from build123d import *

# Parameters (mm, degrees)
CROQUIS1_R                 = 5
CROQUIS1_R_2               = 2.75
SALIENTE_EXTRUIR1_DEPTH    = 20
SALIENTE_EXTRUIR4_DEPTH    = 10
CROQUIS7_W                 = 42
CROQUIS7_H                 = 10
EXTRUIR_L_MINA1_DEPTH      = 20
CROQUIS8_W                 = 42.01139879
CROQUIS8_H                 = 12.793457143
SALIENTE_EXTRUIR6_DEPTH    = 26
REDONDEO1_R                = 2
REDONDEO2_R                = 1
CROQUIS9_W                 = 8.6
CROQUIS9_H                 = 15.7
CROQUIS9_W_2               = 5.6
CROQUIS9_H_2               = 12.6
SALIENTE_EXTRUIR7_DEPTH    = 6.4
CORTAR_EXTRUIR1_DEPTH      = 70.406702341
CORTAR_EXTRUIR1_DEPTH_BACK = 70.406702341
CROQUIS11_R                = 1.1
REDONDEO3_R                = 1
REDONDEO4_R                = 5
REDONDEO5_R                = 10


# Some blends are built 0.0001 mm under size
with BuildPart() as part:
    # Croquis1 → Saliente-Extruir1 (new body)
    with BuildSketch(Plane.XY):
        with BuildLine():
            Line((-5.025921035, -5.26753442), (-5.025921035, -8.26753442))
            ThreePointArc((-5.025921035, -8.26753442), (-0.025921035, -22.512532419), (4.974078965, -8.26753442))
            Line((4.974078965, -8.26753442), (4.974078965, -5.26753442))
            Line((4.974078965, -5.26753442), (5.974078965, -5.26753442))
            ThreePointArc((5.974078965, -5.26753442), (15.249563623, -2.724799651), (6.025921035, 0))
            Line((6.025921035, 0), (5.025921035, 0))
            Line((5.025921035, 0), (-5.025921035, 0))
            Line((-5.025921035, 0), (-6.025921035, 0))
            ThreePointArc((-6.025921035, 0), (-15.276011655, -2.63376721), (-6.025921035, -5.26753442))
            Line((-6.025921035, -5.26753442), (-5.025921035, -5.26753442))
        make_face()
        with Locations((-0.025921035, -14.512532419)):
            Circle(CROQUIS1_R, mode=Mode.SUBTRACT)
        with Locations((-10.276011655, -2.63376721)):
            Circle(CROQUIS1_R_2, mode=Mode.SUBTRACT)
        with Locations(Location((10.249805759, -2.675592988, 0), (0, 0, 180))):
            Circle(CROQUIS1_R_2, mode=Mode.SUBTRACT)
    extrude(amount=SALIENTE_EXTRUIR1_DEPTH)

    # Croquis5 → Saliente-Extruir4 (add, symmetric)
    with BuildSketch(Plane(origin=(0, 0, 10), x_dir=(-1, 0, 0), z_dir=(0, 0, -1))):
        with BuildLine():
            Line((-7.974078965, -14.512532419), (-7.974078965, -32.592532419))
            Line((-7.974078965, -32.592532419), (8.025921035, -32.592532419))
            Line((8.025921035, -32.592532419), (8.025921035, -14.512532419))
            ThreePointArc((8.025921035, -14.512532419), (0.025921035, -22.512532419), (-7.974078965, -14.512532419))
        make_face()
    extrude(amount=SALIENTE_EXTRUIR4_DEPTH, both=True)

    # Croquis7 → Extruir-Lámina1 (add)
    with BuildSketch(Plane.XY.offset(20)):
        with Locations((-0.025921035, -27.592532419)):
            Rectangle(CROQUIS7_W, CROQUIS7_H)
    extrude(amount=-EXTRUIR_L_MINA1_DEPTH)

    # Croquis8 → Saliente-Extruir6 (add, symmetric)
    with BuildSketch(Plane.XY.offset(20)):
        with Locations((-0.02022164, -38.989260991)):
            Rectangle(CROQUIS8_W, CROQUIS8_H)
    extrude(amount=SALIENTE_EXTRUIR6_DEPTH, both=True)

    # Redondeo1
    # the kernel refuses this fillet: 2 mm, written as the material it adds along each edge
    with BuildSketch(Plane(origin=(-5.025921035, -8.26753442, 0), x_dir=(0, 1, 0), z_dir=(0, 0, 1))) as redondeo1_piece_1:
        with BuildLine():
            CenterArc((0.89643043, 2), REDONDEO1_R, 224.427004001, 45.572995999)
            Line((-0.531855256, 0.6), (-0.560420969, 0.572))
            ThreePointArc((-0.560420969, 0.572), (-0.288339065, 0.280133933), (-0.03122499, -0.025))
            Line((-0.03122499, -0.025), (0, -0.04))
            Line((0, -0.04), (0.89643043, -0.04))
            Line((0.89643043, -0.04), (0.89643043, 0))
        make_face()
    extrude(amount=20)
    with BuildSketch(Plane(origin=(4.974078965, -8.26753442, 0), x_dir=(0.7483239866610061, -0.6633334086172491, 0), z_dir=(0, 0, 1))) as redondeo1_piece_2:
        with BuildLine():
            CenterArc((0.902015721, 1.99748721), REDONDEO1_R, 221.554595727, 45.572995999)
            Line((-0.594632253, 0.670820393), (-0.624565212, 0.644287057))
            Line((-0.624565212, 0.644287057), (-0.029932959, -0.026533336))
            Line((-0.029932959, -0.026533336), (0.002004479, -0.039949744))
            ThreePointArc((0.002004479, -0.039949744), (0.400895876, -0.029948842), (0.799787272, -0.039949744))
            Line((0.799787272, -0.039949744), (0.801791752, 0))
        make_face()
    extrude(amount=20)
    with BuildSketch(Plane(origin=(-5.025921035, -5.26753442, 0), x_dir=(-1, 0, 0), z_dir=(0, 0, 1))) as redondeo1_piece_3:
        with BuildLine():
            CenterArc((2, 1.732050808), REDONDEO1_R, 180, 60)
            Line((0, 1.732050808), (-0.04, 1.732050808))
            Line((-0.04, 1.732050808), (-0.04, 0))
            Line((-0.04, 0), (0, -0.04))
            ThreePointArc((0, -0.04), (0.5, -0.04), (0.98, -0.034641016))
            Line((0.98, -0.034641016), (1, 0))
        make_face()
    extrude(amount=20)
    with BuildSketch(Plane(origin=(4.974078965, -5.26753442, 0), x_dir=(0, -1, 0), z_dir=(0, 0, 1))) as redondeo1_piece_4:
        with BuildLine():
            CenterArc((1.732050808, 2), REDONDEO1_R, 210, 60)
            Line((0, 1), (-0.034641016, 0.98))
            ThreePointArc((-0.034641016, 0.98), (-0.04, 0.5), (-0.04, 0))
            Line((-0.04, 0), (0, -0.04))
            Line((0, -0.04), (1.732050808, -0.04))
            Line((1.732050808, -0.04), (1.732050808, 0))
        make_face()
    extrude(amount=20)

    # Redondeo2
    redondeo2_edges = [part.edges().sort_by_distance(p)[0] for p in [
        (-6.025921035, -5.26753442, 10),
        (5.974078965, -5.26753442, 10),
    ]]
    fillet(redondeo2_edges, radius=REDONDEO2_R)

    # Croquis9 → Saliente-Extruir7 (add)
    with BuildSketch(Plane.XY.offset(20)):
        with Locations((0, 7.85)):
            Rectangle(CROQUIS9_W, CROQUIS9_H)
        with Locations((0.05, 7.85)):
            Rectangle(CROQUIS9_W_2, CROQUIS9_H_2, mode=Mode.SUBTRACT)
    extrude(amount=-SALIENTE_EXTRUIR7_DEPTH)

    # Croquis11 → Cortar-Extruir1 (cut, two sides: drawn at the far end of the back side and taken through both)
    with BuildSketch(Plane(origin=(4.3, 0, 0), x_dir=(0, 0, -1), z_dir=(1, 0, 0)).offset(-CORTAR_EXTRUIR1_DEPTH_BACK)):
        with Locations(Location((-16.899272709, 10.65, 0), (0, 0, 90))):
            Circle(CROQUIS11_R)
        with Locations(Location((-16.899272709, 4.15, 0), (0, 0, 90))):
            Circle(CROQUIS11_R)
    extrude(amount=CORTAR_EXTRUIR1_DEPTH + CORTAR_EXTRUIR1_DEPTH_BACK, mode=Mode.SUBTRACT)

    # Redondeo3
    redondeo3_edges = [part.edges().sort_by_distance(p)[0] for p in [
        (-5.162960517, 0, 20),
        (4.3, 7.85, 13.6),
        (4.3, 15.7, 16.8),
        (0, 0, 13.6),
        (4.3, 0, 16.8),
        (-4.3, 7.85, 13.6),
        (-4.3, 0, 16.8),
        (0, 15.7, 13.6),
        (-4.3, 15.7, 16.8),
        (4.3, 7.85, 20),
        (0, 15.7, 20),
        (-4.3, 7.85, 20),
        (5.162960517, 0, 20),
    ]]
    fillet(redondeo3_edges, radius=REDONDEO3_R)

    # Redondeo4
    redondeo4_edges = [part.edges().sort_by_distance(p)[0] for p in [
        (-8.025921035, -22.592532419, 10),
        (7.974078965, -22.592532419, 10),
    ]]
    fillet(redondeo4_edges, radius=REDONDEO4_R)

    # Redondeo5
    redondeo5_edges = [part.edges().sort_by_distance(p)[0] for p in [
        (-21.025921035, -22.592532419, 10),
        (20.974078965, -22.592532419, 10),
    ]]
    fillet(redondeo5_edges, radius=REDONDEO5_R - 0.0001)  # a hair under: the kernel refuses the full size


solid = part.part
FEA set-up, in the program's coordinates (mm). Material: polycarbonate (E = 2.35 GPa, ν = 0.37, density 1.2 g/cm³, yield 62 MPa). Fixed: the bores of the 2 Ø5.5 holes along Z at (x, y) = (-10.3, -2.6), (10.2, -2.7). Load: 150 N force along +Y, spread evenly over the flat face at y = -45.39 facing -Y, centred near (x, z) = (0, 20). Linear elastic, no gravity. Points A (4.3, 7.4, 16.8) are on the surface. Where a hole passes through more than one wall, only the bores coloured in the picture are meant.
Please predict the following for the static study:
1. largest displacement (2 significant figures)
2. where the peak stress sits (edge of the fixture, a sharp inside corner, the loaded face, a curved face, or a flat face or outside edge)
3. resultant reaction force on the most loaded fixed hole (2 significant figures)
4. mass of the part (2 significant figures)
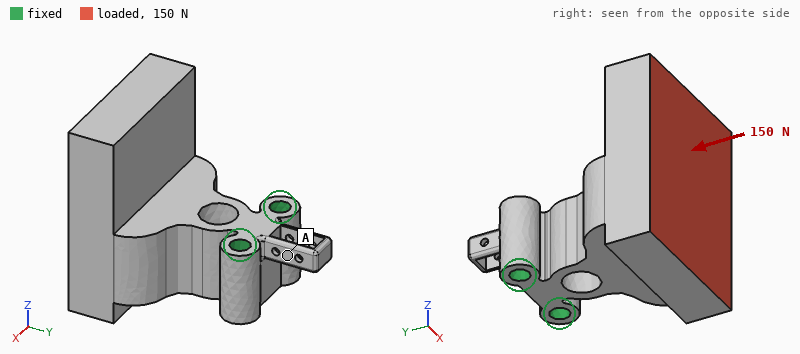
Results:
0.26 mm
a curved face
77 N
51 g
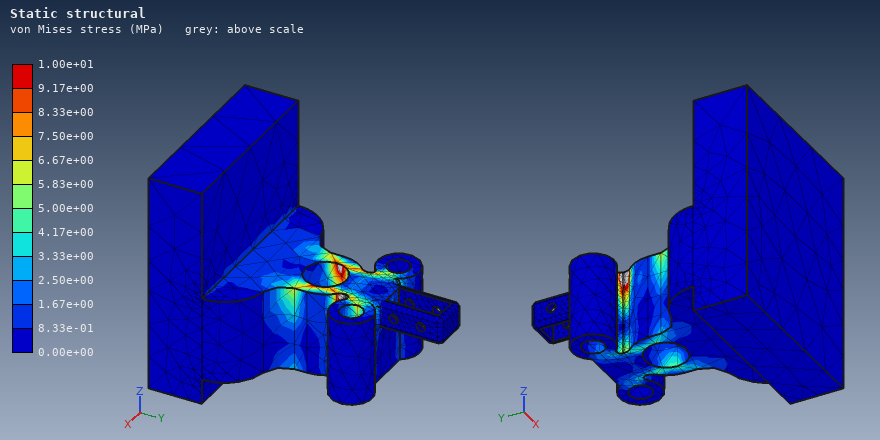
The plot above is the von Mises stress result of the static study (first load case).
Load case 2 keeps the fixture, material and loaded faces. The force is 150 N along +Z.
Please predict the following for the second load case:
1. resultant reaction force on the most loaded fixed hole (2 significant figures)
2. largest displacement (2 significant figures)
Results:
77 N
0.80 mm
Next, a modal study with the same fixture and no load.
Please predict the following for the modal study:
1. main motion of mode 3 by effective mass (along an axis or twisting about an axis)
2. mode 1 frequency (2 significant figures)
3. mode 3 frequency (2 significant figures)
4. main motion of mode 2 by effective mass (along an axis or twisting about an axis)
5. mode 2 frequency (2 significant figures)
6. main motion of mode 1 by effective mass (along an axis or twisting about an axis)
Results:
twisting about Y
340 Hz
680 Hz
along Z
440 Hz
along X
